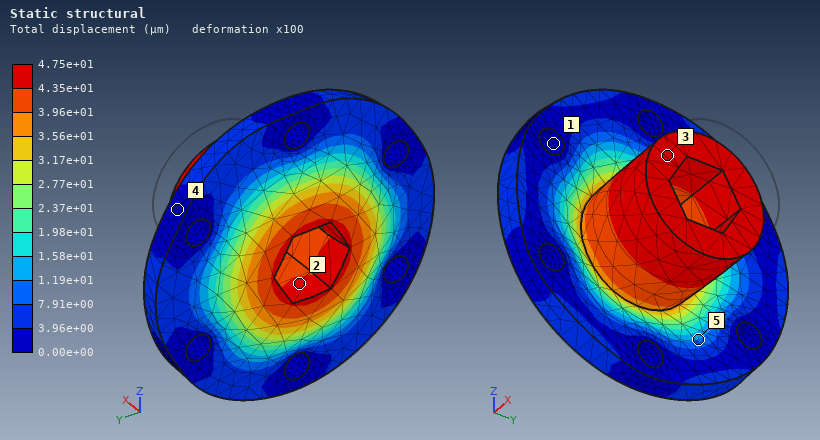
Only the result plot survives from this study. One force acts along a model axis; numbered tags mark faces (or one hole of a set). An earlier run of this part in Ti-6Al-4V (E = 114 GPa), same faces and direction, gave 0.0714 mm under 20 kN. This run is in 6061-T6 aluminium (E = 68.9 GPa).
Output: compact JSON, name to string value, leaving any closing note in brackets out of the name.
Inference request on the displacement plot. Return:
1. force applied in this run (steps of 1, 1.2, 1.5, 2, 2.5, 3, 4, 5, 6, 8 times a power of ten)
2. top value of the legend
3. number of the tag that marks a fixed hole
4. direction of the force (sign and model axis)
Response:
{"force applied in this run": "8 kN", "top value of the legend": "4.75e+01 µm", "number of the tag that marks a fixed hole": "1", "direction of the force": "-X"}
